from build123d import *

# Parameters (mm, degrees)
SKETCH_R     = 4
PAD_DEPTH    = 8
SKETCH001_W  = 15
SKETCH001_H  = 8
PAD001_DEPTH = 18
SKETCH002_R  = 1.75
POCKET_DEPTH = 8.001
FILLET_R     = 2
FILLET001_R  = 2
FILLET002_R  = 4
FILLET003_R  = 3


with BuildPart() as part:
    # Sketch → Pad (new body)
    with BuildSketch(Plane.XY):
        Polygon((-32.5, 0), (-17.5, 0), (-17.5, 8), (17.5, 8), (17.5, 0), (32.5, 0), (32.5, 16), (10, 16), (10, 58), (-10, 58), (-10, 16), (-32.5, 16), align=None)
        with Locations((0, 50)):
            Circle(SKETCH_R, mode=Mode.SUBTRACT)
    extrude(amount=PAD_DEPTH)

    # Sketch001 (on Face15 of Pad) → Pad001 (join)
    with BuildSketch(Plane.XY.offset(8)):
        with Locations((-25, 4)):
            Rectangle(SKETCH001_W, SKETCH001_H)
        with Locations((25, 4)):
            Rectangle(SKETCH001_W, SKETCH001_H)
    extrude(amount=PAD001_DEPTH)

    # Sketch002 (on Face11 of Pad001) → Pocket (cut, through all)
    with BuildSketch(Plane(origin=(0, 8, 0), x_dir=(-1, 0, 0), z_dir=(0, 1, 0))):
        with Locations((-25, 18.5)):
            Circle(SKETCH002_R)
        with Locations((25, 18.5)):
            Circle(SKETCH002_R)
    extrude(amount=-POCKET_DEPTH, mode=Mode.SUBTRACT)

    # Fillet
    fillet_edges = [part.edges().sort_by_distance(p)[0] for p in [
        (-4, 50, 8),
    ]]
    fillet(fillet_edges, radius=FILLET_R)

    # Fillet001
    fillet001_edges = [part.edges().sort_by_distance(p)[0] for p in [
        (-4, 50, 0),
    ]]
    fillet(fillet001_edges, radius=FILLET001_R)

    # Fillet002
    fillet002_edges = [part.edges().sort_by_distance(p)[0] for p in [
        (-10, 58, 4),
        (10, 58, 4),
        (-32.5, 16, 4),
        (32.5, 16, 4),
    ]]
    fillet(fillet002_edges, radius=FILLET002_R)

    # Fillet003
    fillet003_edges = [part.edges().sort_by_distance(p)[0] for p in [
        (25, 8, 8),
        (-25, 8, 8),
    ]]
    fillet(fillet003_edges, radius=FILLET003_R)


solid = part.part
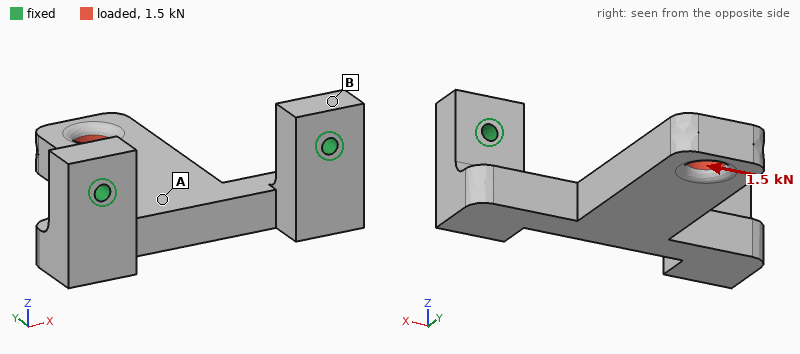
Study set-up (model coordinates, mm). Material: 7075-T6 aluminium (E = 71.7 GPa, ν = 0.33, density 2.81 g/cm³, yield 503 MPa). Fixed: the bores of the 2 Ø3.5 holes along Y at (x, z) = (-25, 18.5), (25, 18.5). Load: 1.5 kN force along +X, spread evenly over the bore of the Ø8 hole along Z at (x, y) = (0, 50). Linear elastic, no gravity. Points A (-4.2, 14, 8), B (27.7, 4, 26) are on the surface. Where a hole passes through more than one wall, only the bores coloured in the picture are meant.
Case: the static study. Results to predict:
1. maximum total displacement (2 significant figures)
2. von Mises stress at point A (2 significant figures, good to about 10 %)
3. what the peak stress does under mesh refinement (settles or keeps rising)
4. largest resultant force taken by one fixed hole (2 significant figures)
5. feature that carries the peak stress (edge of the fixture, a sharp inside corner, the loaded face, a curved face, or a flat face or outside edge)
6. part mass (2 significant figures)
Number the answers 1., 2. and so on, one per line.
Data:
1. 0.31 mm
2. 42 MPa
3. keeps rising
4. 1.7 kN
5. edge of the fixture
6. 46 g
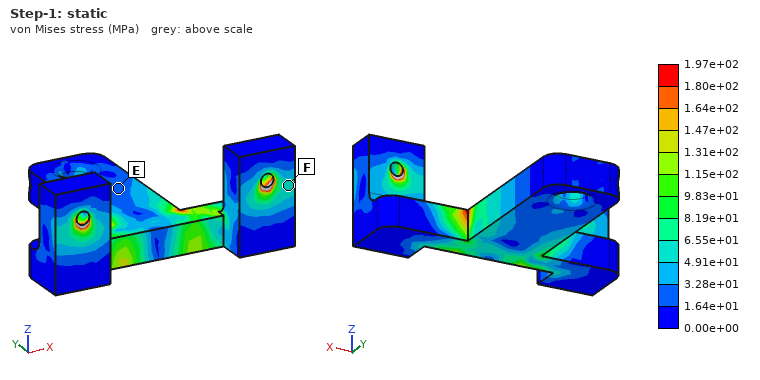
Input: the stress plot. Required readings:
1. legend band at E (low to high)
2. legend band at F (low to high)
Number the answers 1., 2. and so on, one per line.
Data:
1. 1.64e+01 to 3.28e+01 MPa
2. 4.91e+01 to 6.55e+01 MPa
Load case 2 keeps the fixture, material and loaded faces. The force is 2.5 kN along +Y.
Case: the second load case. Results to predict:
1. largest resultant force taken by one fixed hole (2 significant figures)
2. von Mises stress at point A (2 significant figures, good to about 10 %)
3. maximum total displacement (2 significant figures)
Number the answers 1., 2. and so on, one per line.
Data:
1. 1.4 kN
2. 29 MPa
3. 0.23 mm
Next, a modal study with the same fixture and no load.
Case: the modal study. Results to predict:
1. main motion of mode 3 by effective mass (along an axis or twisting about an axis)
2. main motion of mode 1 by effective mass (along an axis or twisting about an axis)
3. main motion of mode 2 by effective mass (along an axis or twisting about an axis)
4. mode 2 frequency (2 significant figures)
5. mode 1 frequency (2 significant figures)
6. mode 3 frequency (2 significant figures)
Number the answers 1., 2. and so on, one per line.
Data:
1. along Y
2. along Z
3. along X
4. 4100 Hz
5. 1500 Hz
6. 5600 Hz
